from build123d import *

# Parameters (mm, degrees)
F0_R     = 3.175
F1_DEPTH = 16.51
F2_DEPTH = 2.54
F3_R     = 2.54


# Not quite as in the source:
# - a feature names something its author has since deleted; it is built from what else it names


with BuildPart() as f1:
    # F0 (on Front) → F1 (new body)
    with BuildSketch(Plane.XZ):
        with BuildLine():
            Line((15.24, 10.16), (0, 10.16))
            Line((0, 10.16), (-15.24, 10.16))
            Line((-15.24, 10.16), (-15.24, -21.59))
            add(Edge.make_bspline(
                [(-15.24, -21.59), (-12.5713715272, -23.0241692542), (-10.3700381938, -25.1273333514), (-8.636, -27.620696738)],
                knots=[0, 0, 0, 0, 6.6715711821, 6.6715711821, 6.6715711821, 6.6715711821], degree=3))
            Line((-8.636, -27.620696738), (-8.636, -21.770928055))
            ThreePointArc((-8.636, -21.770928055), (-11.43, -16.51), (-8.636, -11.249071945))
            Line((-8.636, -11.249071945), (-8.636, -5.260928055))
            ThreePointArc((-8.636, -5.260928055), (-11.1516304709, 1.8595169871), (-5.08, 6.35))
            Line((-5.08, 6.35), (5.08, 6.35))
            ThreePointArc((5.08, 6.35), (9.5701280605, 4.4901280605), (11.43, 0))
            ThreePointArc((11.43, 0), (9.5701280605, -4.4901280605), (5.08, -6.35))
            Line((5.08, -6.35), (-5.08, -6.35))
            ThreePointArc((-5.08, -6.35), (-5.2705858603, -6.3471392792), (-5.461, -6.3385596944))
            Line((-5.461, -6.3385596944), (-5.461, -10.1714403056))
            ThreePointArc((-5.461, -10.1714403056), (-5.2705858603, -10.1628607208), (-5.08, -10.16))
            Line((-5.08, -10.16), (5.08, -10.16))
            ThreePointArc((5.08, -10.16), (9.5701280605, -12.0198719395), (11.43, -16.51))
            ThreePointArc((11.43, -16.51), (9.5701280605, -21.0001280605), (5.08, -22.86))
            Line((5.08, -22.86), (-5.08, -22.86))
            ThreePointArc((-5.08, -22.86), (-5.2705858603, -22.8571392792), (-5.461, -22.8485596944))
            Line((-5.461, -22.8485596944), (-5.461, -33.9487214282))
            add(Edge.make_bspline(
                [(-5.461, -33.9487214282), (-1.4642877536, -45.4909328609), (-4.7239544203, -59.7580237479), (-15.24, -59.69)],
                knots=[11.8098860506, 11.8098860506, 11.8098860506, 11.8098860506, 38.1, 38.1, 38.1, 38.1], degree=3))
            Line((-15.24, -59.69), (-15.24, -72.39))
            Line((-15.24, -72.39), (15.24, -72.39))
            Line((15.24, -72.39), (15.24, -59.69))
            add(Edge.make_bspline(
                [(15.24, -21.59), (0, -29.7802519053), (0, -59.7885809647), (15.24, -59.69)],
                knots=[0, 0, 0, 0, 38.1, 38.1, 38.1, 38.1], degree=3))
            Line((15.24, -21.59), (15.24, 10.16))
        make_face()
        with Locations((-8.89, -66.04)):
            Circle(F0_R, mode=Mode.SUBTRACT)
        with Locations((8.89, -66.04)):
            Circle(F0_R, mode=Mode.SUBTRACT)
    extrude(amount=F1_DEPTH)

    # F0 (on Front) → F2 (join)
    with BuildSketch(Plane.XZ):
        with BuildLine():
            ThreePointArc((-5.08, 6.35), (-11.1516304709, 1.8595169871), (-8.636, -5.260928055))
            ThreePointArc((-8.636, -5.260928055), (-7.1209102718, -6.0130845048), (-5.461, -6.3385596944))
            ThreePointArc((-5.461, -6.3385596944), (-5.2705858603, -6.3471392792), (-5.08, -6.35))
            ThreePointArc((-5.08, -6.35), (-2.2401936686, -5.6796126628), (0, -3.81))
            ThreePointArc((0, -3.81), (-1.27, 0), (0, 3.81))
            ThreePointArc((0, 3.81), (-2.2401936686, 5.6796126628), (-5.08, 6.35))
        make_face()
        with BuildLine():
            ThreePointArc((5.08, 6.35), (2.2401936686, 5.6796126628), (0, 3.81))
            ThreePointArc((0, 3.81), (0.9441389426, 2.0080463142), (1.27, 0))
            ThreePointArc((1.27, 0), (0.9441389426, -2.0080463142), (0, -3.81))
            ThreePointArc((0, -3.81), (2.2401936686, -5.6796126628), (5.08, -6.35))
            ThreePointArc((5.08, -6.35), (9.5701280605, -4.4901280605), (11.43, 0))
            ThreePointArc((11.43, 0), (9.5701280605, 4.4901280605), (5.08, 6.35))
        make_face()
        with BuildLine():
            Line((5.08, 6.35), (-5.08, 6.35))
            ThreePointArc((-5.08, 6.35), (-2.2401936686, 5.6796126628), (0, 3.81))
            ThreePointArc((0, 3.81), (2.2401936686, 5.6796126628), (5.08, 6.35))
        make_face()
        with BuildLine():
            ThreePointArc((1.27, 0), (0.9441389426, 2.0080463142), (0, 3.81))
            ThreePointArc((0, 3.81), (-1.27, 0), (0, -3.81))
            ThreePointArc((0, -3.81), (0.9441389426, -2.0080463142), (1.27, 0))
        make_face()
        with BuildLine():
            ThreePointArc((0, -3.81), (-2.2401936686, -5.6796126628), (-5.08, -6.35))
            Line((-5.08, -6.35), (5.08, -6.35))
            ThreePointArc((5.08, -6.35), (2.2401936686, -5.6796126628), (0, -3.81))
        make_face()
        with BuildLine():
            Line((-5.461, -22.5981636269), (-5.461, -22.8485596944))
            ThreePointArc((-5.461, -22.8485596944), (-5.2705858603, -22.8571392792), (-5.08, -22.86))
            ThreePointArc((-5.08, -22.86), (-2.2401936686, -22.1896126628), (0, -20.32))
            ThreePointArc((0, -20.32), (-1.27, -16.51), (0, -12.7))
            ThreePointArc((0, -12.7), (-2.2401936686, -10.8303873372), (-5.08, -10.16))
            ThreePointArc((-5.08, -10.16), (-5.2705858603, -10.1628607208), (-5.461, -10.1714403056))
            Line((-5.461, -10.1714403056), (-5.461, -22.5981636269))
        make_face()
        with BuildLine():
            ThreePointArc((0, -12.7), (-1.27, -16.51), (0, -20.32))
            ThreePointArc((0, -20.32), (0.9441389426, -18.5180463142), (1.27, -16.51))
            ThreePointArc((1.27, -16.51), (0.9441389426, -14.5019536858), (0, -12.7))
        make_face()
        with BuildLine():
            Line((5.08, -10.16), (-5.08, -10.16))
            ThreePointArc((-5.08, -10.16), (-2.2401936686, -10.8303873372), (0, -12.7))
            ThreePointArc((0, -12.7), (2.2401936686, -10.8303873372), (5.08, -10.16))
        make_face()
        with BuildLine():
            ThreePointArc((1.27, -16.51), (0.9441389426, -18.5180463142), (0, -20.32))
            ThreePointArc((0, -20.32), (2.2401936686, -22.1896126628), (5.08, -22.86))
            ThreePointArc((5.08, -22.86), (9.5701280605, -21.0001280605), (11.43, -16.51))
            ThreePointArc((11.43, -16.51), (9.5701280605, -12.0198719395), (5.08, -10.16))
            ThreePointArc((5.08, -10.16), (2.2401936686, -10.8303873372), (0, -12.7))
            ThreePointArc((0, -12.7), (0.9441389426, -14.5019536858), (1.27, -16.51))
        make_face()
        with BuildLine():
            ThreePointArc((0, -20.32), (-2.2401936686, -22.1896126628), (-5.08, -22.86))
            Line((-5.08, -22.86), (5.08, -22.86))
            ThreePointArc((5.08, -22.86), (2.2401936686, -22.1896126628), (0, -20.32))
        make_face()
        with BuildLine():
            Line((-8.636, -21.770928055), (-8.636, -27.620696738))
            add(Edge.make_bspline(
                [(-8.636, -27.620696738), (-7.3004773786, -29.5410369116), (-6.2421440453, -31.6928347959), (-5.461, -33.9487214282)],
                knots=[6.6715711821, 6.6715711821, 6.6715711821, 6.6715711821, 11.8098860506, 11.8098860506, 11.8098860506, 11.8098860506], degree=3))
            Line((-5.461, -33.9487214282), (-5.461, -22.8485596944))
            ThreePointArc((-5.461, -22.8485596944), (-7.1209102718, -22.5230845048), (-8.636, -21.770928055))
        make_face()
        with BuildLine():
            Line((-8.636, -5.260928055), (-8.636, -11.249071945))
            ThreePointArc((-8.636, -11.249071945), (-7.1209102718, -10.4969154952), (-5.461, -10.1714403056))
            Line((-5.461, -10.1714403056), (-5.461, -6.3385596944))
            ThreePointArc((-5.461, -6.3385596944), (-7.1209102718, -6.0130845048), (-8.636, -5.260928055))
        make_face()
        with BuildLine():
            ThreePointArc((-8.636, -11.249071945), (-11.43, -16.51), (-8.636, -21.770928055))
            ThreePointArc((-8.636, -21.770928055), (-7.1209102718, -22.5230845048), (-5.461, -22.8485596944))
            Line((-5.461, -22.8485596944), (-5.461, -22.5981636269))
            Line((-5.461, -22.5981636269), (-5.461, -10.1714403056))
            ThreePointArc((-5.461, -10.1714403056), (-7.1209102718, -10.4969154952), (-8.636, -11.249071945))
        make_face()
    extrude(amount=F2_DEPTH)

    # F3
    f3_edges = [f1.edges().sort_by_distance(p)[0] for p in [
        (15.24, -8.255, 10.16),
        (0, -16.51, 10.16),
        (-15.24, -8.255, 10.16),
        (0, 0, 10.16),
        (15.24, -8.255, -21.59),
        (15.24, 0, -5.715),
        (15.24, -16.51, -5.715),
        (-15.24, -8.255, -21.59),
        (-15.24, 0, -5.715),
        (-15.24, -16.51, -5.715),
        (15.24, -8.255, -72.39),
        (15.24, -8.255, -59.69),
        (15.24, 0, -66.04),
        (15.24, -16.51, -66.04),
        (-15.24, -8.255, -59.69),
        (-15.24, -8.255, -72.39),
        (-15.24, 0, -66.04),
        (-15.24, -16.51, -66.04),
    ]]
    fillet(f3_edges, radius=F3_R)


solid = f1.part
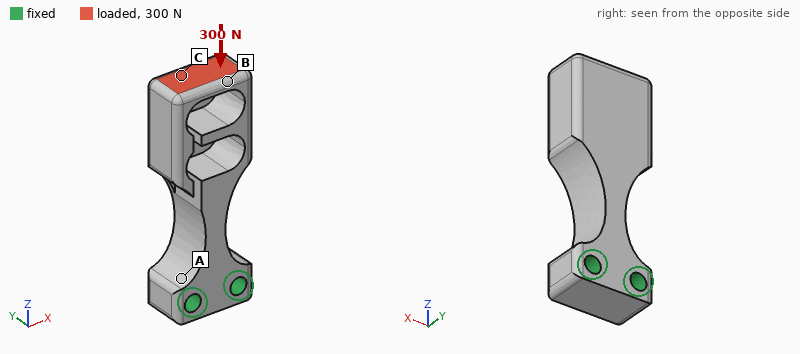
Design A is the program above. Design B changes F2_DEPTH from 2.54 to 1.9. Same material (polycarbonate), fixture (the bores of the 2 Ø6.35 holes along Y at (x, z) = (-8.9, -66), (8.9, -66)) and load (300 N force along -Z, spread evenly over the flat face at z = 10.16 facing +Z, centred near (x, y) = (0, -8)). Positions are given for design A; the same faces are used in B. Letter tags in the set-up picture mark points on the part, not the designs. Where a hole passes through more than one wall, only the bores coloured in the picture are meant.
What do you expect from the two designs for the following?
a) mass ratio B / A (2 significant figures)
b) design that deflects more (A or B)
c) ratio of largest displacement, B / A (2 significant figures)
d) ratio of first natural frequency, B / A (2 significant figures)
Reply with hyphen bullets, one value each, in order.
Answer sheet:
- 0.98
- B
- 1.2
- 1.0
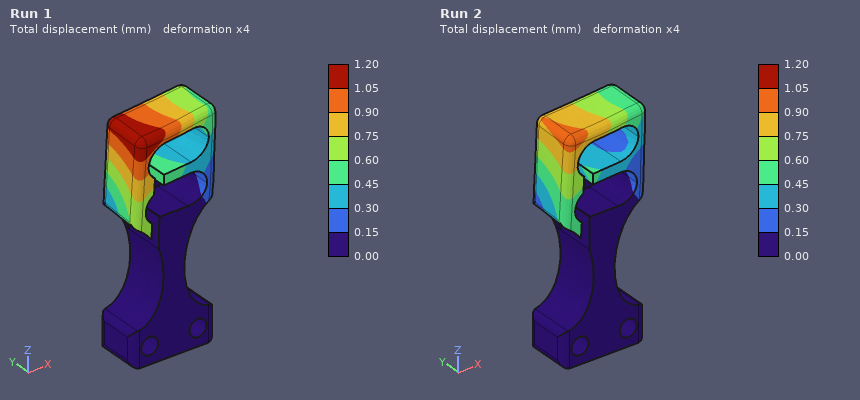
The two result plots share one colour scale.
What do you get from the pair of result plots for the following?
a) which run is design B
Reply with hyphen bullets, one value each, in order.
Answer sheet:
- Run 1
